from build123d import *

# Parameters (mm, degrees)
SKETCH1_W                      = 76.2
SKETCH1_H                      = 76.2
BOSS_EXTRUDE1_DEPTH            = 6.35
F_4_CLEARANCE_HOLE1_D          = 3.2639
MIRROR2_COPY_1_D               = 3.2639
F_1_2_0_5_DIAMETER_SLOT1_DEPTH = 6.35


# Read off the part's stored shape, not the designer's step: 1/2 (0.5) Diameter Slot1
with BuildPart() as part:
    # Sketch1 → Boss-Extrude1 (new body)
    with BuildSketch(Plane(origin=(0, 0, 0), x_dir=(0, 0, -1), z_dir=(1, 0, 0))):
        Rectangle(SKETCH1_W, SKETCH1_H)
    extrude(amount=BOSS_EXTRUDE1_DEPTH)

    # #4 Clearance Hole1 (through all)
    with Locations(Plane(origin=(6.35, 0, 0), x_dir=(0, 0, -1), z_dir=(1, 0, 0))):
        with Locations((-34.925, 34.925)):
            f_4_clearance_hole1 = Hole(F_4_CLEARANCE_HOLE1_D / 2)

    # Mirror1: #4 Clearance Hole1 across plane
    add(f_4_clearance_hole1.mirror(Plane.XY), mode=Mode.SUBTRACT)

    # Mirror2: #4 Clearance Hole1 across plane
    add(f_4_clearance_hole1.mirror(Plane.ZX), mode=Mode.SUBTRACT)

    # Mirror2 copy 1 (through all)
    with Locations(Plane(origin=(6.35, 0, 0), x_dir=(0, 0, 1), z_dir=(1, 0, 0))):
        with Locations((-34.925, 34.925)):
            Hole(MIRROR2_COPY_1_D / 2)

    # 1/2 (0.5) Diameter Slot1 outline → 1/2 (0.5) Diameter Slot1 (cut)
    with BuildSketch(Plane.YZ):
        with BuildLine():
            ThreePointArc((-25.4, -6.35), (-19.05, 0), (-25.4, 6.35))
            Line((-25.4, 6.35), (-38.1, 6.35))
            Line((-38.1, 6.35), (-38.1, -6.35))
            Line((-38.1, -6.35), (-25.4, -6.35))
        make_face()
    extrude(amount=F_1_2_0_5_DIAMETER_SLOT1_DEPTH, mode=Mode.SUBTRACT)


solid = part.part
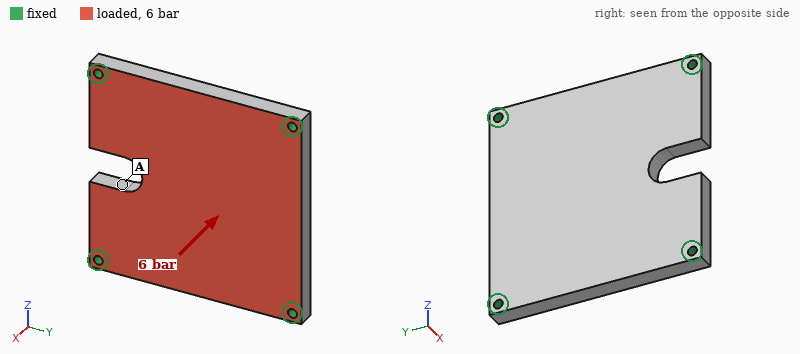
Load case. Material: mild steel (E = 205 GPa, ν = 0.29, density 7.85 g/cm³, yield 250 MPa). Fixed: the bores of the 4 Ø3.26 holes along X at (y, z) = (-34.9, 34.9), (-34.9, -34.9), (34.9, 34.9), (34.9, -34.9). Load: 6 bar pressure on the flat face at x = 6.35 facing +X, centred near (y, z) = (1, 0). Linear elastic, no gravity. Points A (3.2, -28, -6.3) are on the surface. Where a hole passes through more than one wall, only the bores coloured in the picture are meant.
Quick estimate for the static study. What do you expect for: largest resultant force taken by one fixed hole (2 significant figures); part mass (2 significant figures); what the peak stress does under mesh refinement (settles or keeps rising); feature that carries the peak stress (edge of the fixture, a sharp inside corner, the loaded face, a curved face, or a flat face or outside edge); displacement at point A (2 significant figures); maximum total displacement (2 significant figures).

860 N
280 g
keeps rising
edge of the fixture
25 µm
32 µm
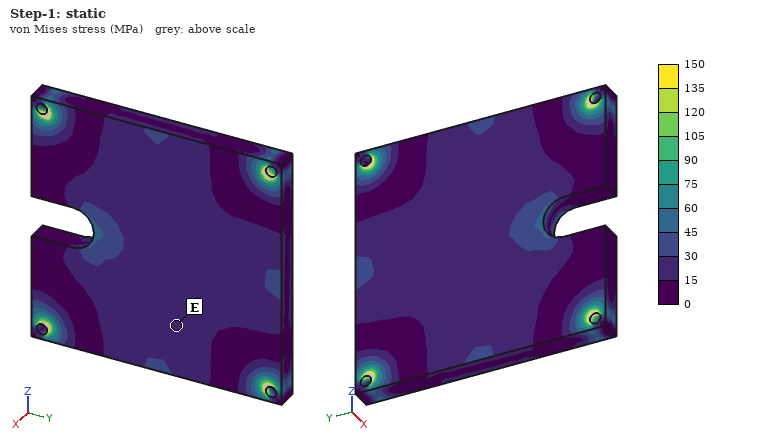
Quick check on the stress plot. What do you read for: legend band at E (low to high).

15 to 30 MPa
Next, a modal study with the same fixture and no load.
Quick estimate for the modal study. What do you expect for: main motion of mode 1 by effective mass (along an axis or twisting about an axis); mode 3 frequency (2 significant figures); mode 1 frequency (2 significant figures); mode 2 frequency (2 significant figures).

along X
6900 Hz
3700 Hz
6700 Hz
